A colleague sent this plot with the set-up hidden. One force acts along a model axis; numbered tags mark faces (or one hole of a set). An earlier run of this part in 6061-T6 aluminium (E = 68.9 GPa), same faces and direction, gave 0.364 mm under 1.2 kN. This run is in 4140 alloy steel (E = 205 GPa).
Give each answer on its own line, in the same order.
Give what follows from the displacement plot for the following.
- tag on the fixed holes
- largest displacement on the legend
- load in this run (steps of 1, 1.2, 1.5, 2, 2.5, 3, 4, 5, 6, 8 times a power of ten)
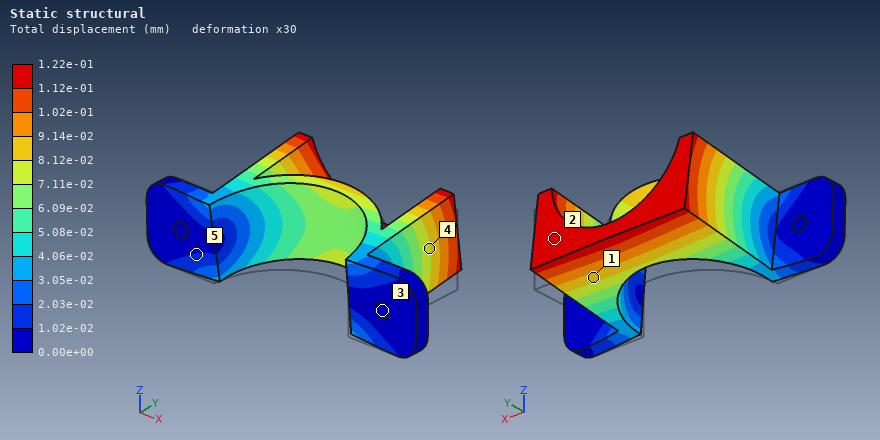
3
1.22e-01 mm
1.2 kN
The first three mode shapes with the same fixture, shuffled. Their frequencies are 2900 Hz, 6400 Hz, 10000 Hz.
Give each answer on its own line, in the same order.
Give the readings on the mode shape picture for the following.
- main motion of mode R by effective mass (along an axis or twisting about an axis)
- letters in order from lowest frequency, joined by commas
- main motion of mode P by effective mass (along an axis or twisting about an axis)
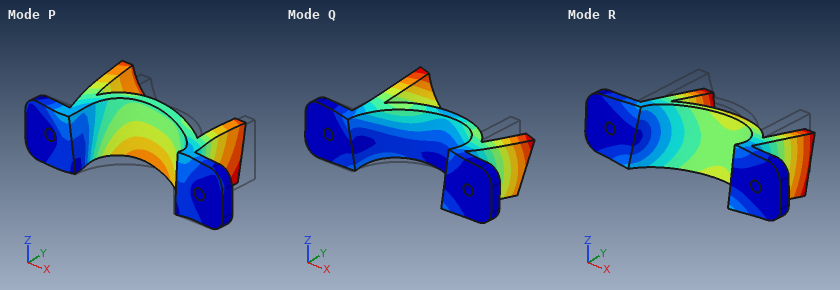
along Z
R, Q, P
along X
